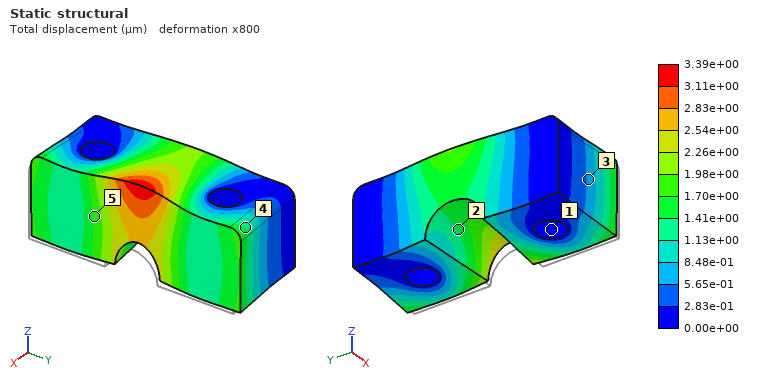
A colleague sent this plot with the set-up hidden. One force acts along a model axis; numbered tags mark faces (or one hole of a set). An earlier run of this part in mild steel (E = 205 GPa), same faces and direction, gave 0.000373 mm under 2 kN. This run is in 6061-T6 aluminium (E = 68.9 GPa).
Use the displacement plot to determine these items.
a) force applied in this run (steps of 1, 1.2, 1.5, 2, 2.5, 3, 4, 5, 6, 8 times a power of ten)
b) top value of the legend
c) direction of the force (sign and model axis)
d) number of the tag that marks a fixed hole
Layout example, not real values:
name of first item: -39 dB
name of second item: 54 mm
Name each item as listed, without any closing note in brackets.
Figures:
force applied in this run: 6 kN
top value of the legend: 3.39e+00 µm
direction of the force: -X
number of the tag that marks a fixed hole: 1
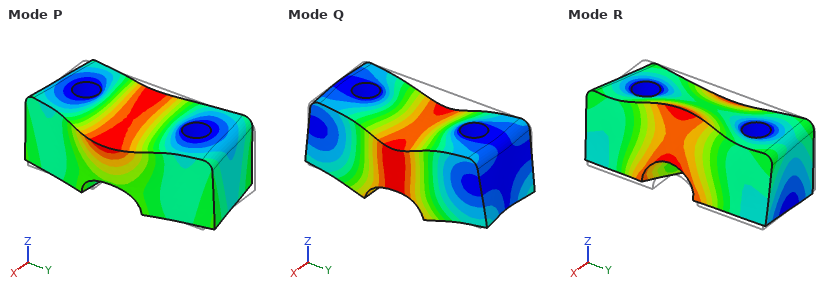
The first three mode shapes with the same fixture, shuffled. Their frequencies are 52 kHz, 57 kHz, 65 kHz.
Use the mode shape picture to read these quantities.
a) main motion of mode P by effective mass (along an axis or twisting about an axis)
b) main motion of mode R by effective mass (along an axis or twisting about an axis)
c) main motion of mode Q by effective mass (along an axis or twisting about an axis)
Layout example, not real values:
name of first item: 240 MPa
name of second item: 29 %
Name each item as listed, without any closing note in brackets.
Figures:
main motion of mode P by effective mass: along X
main motion of mode R by effective mass: twisting about Y
main motion of mode Q by effective mass: along Z
